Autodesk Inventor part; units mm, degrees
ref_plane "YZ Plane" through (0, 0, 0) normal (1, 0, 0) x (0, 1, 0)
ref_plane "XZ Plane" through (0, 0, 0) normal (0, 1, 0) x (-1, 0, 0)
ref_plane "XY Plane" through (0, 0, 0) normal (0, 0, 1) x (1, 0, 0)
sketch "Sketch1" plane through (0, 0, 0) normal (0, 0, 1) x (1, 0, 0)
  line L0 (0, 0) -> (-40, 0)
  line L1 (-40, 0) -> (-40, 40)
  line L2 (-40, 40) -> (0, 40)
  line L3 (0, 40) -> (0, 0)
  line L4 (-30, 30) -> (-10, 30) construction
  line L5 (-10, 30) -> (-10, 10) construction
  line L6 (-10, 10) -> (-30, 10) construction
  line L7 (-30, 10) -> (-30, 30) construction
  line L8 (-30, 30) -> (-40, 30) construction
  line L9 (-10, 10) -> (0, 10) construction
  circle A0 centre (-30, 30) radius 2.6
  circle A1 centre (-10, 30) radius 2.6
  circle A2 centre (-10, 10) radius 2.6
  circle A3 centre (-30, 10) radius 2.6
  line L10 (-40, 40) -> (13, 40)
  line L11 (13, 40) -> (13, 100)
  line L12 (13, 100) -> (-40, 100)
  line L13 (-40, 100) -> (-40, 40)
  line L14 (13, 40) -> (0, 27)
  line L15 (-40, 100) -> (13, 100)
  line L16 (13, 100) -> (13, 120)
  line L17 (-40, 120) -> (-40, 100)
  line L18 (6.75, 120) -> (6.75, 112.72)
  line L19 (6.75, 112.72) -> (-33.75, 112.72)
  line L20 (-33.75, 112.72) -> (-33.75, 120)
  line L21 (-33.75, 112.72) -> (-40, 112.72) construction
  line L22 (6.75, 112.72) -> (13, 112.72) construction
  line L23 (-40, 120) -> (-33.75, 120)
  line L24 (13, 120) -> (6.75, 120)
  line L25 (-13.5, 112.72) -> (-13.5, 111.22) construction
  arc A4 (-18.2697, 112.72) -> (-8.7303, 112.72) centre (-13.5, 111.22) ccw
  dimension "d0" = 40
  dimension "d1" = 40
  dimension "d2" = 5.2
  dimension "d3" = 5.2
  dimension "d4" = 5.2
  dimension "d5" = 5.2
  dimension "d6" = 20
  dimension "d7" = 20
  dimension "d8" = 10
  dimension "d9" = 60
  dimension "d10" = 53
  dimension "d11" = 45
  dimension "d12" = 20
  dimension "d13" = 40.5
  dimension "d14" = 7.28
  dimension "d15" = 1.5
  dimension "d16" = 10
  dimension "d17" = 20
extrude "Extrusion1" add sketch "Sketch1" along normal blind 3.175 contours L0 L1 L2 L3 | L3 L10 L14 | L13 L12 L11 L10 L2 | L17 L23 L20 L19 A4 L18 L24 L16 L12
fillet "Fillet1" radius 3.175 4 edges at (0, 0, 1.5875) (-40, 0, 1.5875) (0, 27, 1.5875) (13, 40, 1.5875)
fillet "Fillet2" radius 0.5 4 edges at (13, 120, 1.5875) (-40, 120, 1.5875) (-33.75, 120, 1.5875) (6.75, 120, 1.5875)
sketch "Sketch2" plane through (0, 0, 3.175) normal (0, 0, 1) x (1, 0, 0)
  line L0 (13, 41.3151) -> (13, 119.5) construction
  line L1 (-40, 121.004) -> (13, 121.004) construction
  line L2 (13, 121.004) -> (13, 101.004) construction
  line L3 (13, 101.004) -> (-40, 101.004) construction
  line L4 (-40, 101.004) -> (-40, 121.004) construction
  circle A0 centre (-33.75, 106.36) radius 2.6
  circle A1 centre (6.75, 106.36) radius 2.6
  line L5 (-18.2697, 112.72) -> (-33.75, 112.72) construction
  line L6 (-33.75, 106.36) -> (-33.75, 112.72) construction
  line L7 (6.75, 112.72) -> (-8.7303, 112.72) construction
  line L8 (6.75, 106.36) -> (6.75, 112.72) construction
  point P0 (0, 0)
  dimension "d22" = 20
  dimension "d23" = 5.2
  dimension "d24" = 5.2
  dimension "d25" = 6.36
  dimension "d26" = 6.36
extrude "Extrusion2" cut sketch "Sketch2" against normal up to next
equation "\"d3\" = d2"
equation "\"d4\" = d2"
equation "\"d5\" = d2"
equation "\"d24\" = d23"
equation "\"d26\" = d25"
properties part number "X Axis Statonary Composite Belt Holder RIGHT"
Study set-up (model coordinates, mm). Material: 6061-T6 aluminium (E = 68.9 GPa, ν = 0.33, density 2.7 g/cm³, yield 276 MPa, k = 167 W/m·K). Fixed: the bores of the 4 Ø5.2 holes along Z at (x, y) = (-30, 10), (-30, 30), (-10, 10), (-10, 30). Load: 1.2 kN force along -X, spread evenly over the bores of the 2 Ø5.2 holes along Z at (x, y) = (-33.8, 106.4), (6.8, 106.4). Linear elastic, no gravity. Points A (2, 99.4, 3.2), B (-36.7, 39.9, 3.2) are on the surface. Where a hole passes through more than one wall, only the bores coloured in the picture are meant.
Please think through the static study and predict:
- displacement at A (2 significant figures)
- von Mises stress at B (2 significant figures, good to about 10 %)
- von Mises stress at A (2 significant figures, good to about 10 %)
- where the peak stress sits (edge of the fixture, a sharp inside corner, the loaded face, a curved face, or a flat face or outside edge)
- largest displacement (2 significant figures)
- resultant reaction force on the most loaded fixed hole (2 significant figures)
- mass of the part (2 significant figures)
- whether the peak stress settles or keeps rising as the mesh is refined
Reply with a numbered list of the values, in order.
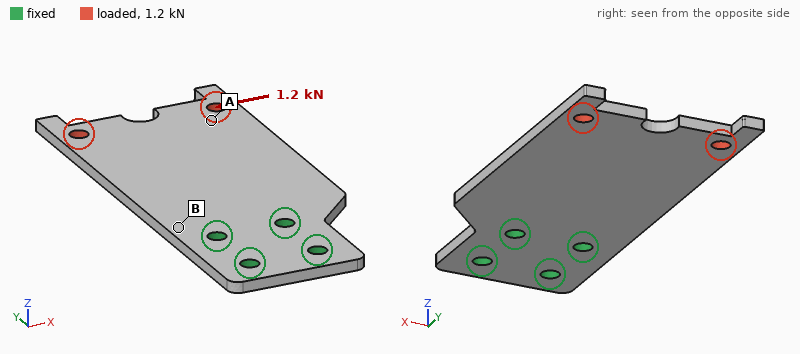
1. 0.14 mm
2. 59 MPa
3. 16 MPa
4. edge of the fixture
5. 0.20 mm
6. 3.1 kN
7. 47 g
8. keeps rising
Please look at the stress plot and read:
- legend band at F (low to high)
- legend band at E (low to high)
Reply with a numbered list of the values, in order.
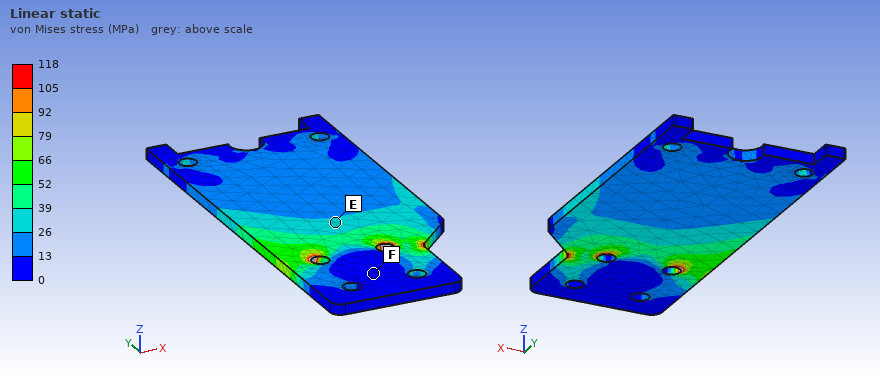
1. 0 to 13 MPa
2. 26 to 39 MPa
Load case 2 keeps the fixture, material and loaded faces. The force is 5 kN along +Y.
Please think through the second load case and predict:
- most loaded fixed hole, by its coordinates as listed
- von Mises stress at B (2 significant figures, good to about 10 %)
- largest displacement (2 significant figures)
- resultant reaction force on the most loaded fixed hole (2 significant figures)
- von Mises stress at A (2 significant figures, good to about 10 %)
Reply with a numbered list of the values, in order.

1. (-10, 30)
2. 16 MPa
3. 81 µm
4. 3.0 kN
5. 48 MPa
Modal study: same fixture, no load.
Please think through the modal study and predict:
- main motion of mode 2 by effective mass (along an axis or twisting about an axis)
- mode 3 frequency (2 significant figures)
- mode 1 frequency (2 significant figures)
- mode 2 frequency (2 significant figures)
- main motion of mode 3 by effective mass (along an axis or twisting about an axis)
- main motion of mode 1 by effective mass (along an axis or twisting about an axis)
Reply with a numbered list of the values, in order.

1. twisting about Y
2. 2200 Hz
3. 380 Hz
4. 1200 Hz
5. along Z
6. along Z
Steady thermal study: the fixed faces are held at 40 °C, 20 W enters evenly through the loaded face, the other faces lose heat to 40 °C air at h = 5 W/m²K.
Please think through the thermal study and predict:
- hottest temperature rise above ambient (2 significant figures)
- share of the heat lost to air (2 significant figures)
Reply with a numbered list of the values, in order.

1. 61 K
2. 7.4 %
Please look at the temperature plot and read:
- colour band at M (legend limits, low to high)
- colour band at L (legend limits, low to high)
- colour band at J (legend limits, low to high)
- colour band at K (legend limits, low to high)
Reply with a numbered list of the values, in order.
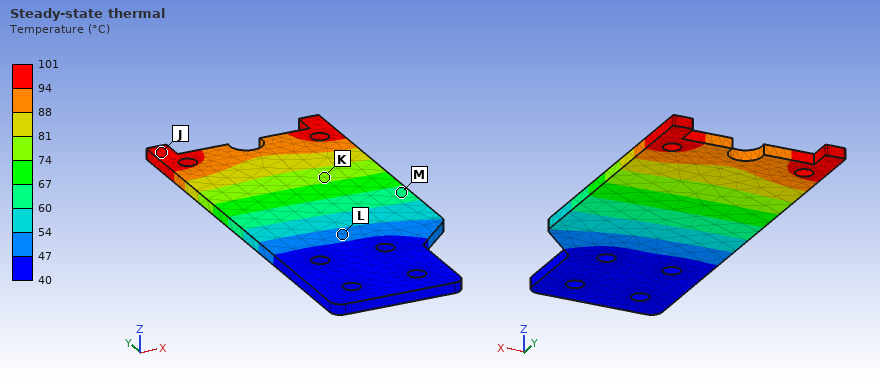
1. 60 to 67 °C
2. 47 to 54 °C
3. 94 to 101 °C
4. 74 to 81 °C
